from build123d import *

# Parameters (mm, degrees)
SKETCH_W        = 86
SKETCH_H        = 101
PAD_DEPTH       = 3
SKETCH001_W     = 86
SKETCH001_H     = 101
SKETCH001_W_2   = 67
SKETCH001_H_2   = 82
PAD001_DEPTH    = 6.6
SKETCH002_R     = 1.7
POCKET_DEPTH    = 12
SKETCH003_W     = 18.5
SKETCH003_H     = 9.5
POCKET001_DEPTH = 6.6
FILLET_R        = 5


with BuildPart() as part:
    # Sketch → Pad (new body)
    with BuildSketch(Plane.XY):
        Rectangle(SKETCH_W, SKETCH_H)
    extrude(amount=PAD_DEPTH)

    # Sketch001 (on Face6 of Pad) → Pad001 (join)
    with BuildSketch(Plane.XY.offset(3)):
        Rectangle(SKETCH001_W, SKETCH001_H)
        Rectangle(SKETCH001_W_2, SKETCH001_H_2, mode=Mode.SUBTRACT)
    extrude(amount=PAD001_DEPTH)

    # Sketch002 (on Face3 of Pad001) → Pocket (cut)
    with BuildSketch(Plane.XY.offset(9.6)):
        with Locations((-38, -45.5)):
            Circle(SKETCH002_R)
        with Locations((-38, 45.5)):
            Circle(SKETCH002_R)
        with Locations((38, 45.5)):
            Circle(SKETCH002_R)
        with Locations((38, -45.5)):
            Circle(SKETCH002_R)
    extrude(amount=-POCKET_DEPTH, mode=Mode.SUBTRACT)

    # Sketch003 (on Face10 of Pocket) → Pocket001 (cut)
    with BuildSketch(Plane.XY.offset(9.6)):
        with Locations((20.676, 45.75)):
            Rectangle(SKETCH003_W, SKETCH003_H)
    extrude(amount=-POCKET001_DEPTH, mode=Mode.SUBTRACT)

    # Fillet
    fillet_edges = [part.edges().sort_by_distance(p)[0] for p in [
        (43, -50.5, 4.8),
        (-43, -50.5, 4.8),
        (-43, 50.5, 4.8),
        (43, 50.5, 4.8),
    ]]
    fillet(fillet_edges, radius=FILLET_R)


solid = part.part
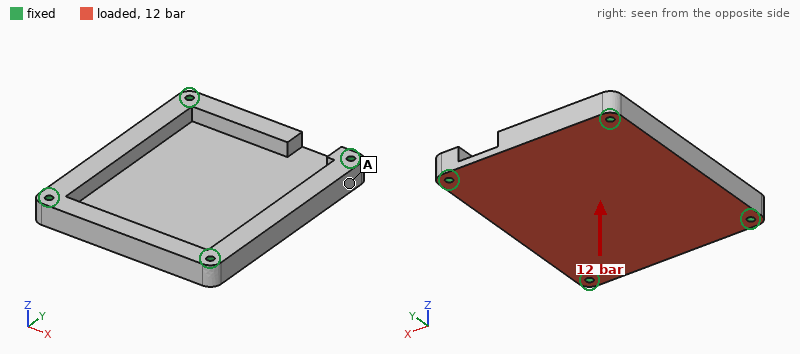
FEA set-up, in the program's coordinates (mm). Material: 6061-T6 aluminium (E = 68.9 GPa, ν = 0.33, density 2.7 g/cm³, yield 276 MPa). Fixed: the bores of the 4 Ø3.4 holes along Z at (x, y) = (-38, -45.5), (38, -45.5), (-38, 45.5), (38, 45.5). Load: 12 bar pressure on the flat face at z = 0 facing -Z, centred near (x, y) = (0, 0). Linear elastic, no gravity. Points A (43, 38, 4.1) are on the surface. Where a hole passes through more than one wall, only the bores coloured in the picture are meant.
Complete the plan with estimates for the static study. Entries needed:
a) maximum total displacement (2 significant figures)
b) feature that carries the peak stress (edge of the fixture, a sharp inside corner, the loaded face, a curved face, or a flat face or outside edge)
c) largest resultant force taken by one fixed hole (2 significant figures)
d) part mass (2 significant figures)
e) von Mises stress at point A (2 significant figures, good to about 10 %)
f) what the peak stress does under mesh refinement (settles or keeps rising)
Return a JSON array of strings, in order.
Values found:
["0.59 mm", "edge of the fixture", "3.8 kN", "120 g", "56 MPa", "keeps rising"]
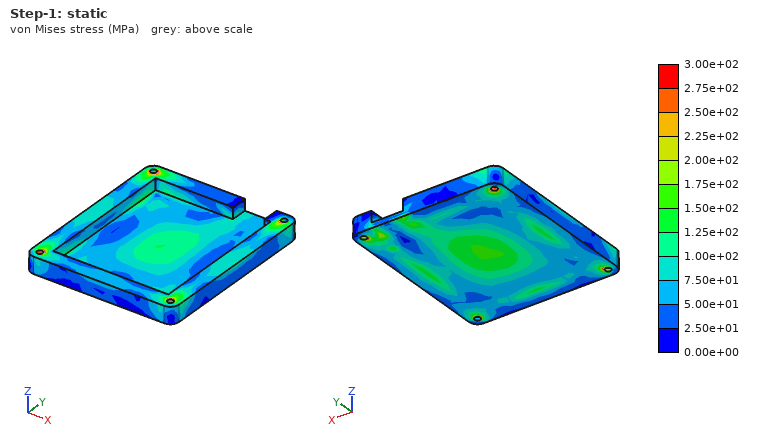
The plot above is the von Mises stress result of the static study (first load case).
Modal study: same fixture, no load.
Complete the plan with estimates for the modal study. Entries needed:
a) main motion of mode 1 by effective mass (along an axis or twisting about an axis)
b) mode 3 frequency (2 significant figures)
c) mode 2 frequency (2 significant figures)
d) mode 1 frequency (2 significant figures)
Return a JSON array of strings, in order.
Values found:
["along Z", "5100 Hz", "5000 Hz", "3200 Hz"]
